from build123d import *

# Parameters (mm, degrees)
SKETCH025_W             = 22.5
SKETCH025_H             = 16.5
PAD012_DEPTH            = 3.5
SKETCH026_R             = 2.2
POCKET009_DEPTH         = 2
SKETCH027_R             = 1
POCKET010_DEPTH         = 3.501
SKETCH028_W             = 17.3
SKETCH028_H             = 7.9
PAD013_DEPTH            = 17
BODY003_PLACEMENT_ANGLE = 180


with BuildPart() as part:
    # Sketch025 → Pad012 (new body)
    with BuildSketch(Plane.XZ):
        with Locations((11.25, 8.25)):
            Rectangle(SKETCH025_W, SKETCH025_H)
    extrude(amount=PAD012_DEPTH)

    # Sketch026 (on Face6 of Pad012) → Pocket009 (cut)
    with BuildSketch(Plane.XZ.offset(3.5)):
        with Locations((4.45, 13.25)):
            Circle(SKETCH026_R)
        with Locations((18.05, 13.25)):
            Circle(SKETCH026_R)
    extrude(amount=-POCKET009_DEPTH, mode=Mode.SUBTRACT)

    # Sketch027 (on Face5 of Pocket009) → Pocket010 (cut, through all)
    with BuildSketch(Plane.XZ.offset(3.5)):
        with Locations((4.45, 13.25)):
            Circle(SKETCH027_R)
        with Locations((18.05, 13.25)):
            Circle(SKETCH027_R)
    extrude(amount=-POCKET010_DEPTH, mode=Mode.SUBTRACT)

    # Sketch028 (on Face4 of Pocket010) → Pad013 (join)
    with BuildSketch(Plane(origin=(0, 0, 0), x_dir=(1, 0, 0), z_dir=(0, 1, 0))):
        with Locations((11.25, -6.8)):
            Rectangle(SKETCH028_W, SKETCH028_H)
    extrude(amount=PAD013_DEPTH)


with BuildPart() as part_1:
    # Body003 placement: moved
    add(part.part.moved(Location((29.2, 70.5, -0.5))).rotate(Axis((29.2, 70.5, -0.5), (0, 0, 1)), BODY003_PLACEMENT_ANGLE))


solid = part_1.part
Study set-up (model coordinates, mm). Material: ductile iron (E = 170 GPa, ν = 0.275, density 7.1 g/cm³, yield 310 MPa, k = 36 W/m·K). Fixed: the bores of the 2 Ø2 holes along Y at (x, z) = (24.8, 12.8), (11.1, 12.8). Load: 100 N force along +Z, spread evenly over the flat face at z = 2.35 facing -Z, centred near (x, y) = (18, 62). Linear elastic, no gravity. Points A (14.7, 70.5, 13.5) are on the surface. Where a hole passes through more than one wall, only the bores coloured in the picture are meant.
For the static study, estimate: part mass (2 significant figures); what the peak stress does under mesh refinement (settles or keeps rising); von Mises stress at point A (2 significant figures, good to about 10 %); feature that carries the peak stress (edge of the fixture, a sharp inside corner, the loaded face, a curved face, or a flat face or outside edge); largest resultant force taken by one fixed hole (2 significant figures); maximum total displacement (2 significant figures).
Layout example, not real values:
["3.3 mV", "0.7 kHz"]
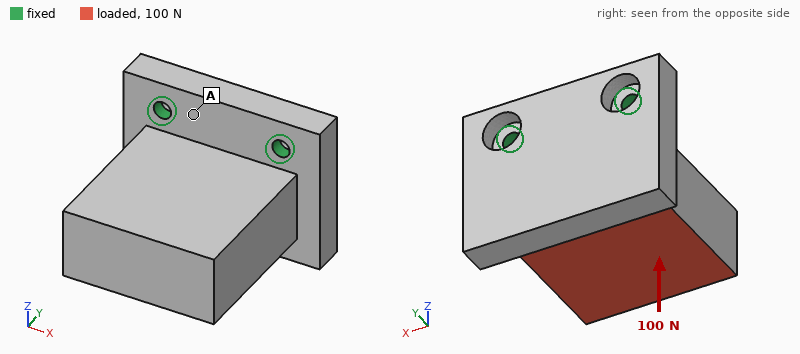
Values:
["25 g", "keeps rising", "14 MPa", "edge of the fixture", "50 N", "22 µm"]
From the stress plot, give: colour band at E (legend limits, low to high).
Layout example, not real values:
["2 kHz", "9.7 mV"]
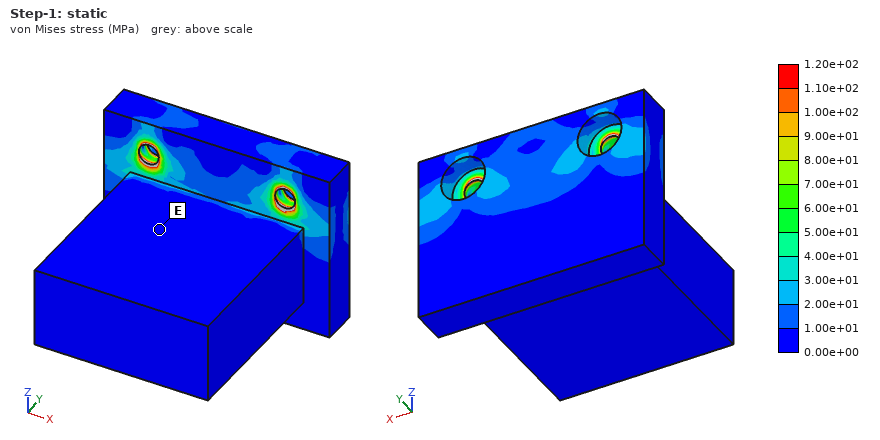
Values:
["0.00e+00 to 1.00e+01 MPa"]
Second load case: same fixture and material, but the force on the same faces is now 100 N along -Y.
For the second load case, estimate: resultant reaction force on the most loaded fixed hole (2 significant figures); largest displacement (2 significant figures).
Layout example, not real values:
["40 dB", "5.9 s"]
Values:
["50 N", "22 µm"]
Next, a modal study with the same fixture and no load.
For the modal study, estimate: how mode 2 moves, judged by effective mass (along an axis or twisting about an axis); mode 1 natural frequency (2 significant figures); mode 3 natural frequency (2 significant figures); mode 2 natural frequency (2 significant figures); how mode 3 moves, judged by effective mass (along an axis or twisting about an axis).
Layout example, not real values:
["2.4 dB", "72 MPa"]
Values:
["along X", "2800 Hz", "17 kHz", "9600 Hz", "along Y"]
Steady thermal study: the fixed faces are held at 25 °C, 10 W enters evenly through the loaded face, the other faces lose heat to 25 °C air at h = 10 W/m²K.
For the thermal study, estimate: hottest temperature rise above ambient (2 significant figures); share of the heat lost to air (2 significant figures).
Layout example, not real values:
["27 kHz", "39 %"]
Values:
["51 K", "5.1 %"]
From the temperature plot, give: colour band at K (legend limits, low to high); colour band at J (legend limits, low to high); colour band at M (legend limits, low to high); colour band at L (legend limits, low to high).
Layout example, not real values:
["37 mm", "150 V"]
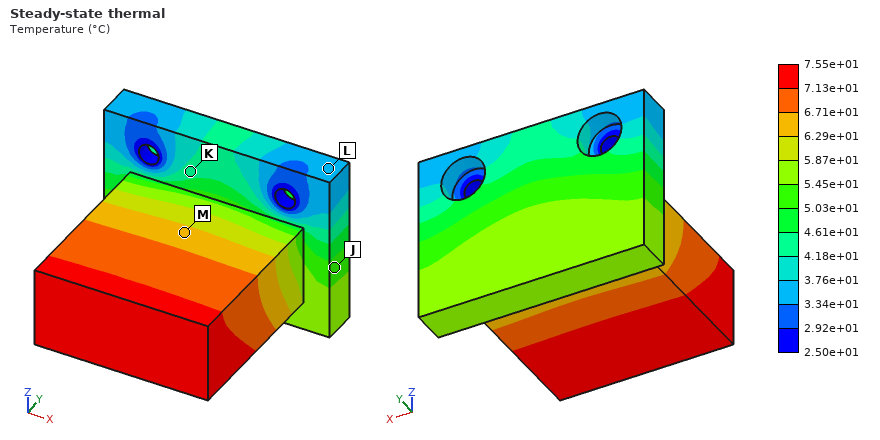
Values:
["4.18e+01 to 4.61e+01 °C", "5.03e+01 to 5.45e+01 °C", "6.29e+01 to 6.71e+01 °C", "3.34e+01 to 3.76e+01 °C"]
